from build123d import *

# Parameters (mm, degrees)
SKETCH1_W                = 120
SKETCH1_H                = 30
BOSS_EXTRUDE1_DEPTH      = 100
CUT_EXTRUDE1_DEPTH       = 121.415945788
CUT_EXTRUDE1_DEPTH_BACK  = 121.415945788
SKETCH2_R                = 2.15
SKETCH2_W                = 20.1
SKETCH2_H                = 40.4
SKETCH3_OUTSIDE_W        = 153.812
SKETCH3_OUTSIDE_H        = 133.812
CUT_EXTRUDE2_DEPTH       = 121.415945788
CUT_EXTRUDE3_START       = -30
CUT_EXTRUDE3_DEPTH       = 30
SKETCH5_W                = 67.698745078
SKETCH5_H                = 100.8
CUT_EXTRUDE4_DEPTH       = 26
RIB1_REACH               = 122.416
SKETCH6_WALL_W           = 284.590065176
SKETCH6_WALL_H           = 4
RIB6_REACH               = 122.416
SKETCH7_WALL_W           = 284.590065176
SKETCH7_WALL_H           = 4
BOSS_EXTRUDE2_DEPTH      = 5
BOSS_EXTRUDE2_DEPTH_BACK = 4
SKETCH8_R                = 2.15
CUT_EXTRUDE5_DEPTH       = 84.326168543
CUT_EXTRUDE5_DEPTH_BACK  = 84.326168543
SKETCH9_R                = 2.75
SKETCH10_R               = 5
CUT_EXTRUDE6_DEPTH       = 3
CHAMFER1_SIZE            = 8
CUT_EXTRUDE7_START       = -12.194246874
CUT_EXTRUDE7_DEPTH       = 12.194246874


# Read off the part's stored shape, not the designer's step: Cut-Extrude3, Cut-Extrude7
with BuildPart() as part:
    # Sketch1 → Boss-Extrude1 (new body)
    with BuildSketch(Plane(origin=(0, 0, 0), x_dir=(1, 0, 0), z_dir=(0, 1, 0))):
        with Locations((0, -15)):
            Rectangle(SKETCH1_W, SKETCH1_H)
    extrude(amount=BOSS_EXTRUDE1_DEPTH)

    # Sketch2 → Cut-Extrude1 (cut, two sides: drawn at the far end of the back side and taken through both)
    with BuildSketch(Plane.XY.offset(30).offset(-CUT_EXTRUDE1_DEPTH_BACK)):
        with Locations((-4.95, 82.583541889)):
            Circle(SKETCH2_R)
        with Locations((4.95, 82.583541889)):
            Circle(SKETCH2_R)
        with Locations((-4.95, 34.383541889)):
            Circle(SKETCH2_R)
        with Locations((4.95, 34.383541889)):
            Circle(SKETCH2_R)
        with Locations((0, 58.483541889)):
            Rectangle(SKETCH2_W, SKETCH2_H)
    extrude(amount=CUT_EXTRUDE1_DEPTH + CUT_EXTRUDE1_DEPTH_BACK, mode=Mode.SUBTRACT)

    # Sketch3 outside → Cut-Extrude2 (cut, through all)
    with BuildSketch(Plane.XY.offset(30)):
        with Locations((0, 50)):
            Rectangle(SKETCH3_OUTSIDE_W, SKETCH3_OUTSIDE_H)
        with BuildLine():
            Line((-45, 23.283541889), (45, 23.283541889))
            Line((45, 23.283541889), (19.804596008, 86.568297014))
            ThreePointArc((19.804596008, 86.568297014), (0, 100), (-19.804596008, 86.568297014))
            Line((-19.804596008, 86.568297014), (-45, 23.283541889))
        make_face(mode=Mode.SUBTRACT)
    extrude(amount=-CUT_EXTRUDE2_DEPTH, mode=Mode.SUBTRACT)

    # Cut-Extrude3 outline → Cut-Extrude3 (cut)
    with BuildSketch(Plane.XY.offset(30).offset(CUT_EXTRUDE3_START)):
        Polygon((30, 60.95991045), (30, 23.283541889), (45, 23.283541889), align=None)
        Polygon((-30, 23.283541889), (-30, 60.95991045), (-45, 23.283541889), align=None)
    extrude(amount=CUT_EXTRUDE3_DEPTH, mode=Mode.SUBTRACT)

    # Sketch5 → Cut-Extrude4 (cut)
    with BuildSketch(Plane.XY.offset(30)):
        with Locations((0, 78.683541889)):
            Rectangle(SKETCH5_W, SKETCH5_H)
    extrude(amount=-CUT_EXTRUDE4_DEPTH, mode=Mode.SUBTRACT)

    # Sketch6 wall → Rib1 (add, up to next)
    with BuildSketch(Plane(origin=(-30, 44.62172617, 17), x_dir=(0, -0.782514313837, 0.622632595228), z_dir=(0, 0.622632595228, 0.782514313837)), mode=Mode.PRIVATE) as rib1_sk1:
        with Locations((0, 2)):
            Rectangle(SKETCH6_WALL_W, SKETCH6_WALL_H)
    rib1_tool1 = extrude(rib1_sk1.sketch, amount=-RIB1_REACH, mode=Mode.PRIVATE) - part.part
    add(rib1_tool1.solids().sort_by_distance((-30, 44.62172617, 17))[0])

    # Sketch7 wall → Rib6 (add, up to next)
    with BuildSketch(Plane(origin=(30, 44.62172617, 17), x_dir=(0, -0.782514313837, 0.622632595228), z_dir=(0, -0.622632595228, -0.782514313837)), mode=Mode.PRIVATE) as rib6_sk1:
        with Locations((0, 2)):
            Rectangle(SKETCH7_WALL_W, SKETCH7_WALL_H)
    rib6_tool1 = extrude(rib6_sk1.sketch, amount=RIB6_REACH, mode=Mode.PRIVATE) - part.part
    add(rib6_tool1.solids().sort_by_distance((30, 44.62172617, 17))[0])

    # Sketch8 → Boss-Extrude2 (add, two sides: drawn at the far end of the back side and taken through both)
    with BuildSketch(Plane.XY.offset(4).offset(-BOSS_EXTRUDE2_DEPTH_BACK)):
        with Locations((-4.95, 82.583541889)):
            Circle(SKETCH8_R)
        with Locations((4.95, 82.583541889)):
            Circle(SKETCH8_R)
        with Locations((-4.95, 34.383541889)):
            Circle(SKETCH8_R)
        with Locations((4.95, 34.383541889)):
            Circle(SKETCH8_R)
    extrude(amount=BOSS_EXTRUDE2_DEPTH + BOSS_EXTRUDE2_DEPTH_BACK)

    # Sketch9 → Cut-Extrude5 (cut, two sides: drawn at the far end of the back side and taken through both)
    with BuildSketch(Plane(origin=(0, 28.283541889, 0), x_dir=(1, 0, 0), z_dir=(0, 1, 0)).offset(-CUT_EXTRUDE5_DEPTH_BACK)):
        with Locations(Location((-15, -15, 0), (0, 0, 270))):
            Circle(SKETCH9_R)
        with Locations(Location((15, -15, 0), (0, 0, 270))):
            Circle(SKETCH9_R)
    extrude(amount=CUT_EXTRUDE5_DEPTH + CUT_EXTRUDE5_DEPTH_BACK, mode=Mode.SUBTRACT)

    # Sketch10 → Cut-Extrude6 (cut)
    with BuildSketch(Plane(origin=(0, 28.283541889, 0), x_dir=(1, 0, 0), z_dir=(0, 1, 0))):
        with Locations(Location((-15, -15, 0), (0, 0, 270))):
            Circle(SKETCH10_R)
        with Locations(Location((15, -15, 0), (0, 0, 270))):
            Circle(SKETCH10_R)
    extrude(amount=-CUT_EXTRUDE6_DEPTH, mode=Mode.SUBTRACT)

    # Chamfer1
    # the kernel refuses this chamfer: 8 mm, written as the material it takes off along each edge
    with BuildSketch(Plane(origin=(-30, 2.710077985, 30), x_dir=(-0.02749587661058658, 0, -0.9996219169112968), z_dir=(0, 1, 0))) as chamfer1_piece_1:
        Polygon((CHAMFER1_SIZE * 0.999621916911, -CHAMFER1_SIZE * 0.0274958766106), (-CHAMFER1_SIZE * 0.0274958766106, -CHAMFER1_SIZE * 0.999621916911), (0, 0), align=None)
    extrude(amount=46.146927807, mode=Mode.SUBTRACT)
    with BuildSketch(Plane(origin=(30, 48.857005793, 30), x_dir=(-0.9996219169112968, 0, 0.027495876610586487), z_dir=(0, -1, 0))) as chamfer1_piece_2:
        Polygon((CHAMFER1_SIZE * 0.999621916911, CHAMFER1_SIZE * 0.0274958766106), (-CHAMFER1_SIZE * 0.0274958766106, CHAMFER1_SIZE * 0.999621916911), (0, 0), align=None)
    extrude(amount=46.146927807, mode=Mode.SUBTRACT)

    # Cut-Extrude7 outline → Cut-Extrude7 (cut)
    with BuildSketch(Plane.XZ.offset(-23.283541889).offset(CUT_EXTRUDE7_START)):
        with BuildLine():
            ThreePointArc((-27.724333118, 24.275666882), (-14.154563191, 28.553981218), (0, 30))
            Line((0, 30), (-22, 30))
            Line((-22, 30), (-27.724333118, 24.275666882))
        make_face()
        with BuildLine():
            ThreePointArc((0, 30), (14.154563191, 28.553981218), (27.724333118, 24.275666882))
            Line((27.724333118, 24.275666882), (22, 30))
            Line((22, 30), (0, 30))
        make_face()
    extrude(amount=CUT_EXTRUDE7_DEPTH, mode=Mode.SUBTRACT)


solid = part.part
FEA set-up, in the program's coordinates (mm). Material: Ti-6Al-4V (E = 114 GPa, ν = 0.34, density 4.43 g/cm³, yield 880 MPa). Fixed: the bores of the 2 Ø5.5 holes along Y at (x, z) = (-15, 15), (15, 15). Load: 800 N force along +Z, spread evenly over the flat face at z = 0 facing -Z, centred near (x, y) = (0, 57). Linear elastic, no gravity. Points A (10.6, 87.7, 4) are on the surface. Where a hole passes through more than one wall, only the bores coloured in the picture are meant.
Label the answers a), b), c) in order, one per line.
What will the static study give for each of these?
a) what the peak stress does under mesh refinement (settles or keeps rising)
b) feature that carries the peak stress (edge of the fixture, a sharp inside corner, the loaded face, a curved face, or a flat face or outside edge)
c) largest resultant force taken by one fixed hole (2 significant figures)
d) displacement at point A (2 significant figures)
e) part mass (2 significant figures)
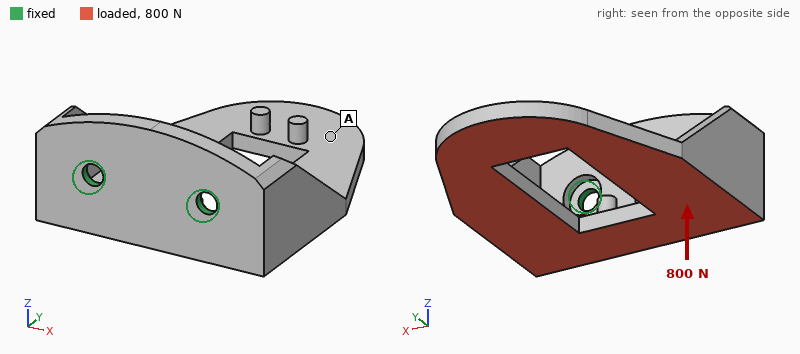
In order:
a) keeps rising
b) edge of the fixture
c) 630 N
d) 0.64 mm
e) 100 g
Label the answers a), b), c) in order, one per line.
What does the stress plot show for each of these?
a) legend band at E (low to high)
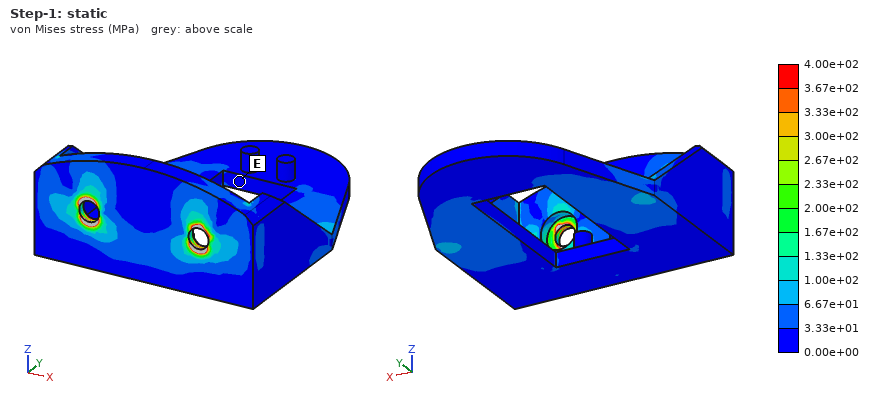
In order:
a) 0.00e+00 to 3.33e+01 MPa
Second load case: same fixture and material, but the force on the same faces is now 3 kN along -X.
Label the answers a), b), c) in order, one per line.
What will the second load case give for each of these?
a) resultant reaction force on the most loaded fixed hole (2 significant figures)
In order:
a) 3.6 kN
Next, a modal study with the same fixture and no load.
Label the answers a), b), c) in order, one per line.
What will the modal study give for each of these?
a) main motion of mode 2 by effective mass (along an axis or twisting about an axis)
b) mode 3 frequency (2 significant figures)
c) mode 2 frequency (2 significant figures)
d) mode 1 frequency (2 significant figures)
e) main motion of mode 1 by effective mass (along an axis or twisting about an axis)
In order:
a) along X
b) 2900 Hz
c) 1800 Hz
d) 840 Hz
e) along Z
